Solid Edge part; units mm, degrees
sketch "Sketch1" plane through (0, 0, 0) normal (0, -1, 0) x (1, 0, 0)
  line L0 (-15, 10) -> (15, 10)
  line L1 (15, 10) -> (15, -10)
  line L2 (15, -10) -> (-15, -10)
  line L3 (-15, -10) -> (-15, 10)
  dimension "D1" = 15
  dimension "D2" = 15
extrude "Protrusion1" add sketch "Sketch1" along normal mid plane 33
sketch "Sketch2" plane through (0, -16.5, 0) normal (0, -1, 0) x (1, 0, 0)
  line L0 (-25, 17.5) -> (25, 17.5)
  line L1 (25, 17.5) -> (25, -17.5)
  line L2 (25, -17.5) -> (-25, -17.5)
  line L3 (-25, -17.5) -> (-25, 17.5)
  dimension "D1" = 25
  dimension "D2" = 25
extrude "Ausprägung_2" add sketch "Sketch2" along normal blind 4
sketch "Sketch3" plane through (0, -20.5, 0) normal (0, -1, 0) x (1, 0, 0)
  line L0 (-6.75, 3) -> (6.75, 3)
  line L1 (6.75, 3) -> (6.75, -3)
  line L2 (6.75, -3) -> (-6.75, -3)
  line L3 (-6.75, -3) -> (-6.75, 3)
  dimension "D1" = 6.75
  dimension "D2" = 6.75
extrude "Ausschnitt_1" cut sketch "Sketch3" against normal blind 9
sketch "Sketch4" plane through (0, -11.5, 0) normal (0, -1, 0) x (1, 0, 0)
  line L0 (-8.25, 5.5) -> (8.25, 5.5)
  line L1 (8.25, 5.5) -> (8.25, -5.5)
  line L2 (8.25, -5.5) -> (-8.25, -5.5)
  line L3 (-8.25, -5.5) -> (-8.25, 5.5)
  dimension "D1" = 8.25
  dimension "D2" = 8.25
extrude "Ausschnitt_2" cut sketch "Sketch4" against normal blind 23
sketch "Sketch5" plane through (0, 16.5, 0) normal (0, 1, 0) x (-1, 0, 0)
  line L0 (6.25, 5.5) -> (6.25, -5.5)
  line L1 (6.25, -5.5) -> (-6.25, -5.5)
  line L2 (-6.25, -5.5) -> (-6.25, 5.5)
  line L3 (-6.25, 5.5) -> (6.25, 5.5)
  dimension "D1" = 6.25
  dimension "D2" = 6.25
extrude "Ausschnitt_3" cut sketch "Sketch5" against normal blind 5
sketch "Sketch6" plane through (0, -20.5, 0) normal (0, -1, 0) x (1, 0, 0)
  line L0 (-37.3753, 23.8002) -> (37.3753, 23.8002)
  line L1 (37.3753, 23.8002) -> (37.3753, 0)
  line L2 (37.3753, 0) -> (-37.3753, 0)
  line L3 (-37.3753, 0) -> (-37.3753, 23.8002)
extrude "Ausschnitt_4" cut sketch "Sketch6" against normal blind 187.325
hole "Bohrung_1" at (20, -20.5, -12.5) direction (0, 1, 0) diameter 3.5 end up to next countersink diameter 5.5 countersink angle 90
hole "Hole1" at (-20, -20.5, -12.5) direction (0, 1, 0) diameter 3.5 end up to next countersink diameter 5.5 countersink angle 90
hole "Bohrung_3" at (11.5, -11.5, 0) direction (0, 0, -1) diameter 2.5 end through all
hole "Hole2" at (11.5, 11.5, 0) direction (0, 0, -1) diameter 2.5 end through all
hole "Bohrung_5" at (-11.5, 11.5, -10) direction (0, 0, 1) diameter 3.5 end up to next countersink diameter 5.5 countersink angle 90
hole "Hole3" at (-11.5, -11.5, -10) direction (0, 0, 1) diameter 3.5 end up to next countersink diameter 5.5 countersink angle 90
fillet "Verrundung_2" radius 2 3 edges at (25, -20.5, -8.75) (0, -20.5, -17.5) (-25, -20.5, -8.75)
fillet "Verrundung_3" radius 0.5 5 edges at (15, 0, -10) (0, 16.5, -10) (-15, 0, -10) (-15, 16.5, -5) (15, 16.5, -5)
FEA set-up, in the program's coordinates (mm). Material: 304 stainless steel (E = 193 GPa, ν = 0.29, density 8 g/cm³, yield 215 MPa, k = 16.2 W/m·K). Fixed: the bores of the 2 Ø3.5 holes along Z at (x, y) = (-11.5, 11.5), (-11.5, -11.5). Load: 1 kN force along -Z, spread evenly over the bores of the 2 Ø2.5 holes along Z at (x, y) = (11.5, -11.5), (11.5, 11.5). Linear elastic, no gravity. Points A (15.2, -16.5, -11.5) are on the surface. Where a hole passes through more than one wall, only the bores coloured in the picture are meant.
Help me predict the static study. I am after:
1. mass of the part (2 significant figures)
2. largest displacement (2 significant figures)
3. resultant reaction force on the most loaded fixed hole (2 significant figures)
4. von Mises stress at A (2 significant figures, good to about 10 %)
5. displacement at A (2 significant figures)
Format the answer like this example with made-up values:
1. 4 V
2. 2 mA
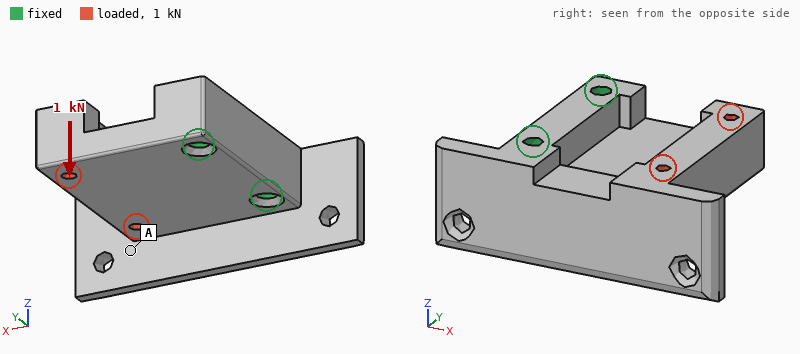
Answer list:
1. 81 g
2. 54 µm
3. 530 N
4. 15 MPa
5. 29 µm
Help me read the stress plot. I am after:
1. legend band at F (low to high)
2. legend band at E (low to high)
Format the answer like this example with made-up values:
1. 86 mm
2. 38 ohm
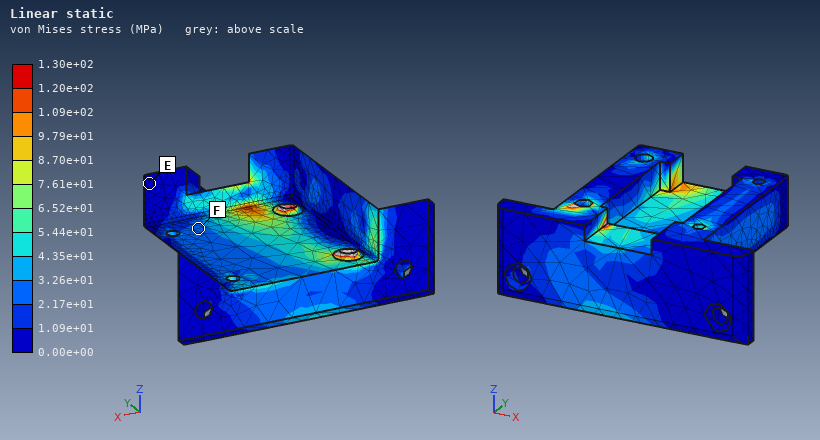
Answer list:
1. 2.17e+01 to 3.26e+01 MPa
2. 0.00e+00 to 1.09e+01 MPa
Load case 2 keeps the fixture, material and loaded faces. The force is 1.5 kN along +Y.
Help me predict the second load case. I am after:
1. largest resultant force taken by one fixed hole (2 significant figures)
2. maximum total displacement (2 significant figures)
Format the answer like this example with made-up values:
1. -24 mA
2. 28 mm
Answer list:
1. 1.5 kN
2. 12 µm
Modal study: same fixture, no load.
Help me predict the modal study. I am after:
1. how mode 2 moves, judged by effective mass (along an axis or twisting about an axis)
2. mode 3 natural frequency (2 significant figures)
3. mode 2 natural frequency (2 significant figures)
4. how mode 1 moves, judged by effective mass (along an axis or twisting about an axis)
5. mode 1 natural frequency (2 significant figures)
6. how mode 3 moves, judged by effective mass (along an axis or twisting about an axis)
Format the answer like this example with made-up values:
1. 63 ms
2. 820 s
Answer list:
1. twisting about X
2. 11 kHz
3. 7600 Hz
4. along Z
5. 4600 Hz
6. along Y
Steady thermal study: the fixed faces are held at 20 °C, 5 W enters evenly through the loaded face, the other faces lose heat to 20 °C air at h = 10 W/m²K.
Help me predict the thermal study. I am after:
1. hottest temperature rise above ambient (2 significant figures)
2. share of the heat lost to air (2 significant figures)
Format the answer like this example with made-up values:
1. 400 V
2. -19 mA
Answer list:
1. 40 K
2. 16 %
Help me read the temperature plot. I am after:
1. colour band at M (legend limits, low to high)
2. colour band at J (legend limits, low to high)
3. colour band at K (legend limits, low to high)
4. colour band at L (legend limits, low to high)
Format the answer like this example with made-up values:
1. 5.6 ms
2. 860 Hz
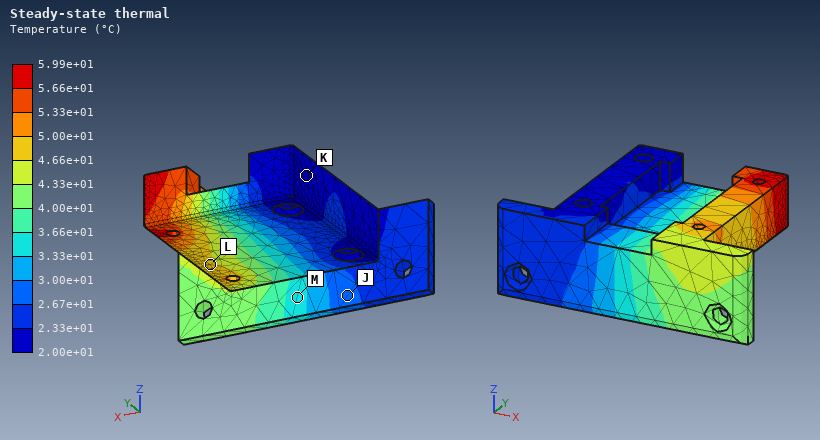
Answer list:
1. 3.33e+01 to 3.66e+01 °C
2. 2.67e+01 to 3.00e+01 °C
3. 2.00e+01 to 2.33e+01 °C
4. 4.66e+01 to 5.00e+01 °C
